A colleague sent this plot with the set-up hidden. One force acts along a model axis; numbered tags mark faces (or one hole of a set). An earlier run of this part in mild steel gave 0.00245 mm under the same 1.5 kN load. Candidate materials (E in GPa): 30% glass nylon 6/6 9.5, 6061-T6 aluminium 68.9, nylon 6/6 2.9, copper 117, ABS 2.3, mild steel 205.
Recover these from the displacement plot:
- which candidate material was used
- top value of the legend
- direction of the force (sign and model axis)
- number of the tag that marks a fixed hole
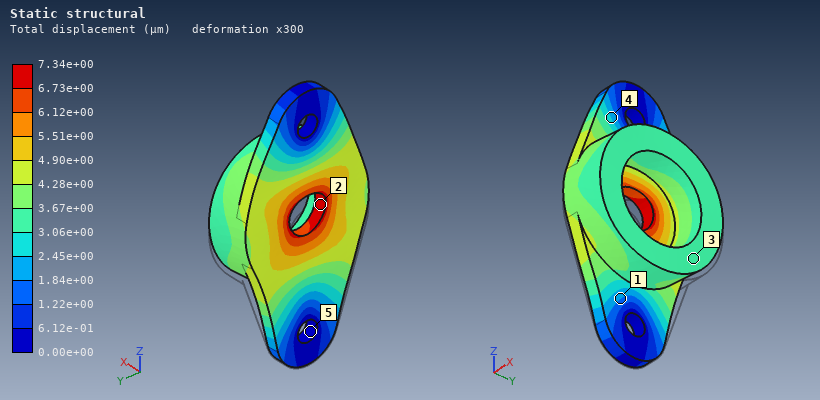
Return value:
6061-T6 aluminium
7.34e+00 µm
+Z
5
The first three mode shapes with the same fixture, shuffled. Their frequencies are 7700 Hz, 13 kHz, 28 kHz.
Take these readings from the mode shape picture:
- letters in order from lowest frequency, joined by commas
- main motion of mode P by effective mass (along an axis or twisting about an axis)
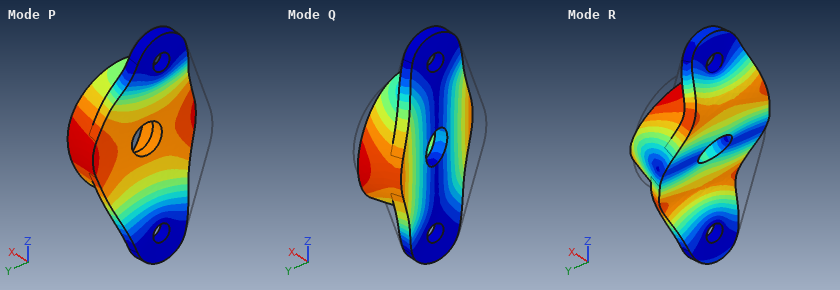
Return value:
Q, P, R
along X
